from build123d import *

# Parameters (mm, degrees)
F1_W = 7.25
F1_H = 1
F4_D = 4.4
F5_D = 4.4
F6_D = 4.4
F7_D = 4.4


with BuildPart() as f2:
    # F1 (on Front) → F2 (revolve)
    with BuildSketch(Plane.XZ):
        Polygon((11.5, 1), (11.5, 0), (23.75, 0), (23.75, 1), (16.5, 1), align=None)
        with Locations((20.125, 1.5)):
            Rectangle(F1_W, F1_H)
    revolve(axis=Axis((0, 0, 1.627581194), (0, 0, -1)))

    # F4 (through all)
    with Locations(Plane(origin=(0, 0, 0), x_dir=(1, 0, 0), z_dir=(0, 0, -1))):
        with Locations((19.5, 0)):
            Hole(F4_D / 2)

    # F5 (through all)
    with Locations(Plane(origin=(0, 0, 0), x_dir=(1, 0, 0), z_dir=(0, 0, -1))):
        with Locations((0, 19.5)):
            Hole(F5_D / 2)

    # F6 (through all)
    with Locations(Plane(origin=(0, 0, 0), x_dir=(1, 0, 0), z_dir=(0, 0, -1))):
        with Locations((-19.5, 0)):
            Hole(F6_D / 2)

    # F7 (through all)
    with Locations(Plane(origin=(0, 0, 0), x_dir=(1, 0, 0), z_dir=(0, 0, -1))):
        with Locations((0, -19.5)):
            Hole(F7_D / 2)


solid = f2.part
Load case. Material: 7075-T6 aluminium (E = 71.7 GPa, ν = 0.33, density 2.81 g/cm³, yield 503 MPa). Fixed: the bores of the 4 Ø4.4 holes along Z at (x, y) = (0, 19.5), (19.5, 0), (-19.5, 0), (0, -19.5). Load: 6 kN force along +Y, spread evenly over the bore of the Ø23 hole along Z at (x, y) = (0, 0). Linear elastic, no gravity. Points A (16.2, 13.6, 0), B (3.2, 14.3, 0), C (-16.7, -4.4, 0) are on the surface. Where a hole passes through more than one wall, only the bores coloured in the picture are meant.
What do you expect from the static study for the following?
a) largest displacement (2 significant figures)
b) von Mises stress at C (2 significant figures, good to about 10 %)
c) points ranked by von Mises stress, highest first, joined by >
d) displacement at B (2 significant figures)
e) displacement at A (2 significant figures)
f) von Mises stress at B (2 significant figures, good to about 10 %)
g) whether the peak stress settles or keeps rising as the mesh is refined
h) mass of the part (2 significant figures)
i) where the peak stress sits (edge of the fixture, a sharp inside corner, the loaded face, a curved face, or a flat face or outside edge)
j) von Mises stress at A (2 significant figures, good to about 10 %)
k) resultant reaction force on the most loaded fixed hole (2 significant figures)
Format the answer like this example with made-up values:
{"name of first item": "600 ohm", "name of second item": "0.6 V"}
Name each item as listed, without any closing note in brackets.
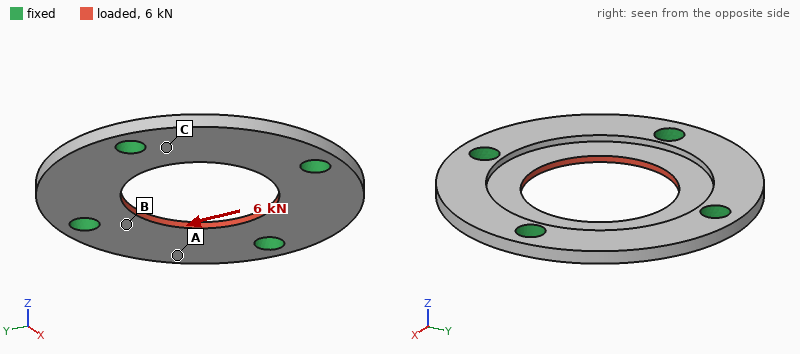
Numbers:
{"largest displacement": "29 µm", "von Mises stress at C": "78 MPa", "points ranked by von Mises stress, highest first, joined by >": "B > C > A", "displacement at B": "13 µm", "displacement at A": "17 µm", "von Mises stress at B": "130 MPa", "whether the peak stress settles or keeps rising as the mesh is refined": "keeps rising", "mass of the part": "6.0 g", "where the peak stress sits": "edge of the fixture", "von Mises stress at A": "39 MPa", "resultant reaction force on the most loaded fixed hole": "1.6 kN"}
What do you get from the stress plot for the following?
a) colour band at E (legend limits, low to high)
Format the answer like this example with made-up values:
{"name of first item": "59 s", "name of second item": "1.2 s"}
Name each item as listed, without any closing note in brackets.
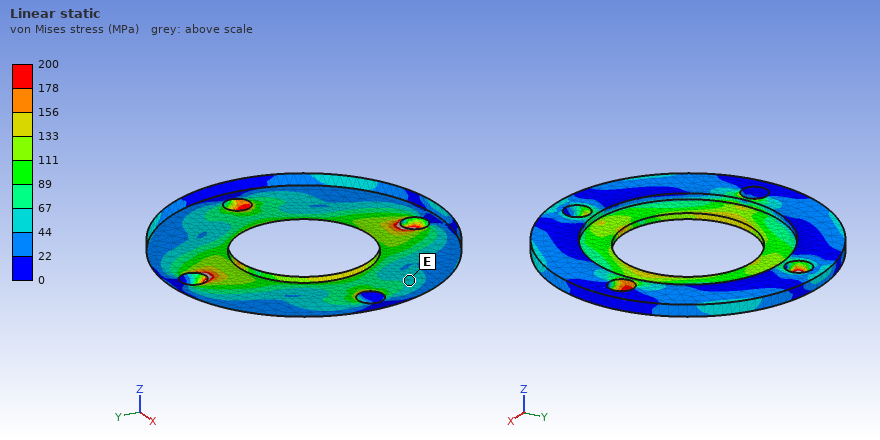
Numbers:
{"colour band at E": "44 to 67 MPa"}
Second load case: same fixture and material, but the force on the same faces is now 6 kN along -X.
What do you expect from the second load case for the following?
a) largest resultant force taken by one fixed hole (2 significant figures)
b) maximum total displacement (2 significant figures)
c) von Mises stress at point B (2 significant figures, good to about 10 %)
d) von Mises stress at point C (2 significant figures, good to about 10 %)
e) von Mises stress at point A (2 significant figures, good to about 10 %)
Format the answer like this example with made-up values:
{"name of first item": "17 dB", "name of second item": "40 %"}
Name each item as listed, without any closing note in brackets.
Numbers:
{"largest resultant force taken by one fixed hole": "1.6 kN", "maximum total displacement": "29 µm", "von Mises stress at point B": "75 MPa", "von Mises stress at point C": "110 MPa", "von Mises stress at point A": "37 MPa"}
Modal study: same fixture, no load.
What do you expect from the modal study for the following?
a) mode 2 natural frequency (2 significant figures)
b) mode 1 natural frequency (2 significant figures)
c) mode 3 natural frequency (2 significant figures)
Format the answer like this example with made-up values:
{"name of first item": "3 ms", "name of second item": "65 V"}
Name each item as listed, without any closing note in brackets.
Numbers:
{"mode 2 natural frequency": "12 kHz", "mode 1 natural frequency": "12 kHz", "mode 3 natural frequency": "12 kHz"}
